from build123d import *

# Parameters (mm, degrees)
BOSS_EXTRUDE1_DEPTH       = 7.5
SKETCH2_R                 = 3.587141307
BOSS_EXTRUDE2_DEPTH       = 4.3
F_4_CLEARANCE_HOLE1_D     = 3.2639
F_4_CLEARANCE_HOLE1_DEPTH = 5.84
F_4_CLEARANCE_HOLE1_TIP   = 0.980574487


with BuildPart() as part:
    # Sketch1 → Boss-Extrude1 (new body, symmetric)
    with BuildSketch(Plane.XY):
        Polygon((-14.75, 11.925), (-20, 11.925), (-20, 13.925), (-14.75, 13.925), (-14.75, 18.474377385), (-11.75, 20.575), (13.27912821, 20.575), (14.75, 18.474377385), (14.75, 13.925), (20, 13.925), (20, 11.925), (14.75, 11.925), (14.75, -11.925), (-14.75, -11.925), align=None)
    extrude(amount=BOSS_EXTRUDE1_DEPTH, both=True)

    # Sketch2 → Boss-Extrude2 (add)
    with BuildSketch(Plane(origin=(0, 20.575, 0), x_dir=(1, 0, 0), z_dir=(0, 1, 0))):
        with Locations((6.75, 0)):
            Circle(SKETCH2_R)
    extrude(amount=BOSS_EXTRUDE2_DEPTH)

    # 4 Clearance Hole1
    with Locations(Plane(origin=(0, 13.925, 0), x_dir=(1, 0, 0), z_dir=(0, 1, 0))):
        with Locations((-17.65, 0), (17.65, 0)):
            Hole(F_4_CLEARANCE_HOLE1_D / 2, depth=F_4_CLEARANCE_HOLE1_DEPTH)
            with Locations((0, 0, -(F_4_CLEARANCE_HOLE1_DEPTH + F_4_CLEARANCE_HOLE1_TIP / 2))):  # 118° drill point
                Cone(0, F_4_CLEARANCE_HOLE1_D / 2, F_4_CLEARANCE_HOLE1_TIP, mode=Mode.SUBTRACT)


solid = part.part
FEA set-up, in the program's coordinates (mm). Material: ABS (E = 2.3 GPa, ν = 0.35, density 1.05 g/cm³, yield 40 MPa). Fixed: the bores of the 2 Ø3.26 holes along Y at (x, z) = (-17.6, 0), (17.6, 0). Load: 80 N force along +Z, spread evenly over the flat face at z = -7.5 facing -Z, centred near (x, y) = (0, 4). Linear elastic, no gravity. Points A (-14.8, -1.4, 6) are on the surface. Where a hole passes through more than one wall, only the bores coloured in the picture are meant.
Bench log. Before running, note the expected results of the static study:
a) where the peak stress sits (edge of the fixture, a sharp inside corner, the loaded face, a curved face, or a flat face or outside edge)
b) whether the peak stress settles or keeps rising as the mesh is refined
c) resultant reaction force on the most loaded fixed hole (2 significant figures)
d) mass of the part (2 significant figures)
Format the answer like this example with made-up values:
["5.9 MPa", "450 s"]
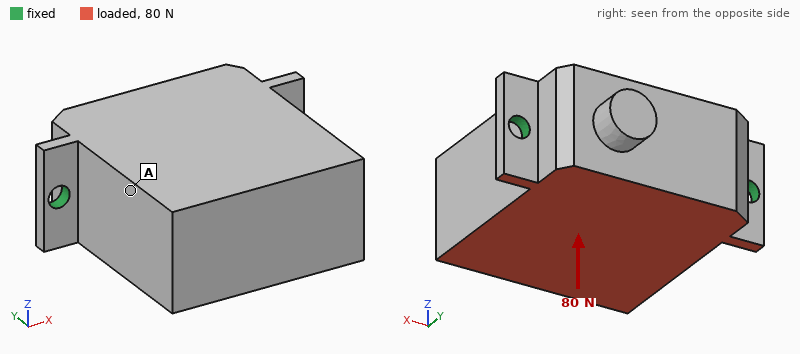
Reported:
["edge of the fixture", "keeps rising", "40 N", "16 g"]
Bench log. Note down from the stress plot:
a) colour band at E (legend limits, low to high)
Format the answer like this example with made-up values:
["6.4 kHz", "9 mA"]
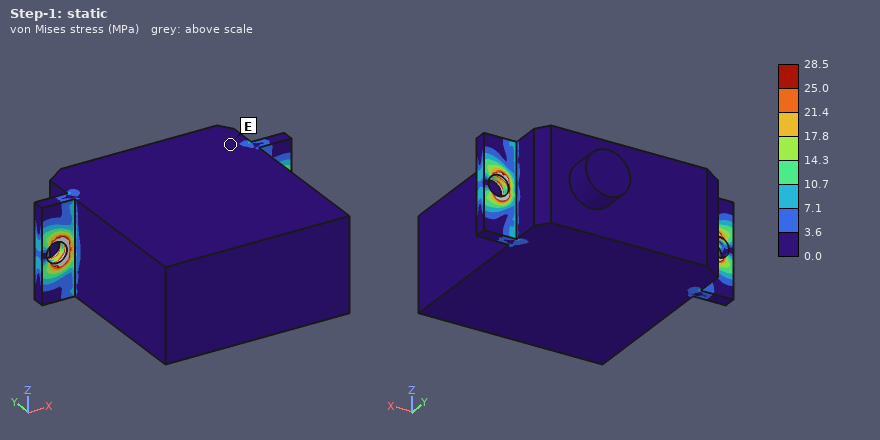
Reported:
["0.0 to 3.6 MPa"]
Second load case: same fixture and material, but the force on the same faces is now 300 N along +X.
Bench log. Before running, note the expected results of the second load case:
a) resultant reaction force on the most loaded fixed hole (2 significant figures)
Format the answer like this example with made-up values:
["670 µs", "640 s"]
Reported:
["180 N"]
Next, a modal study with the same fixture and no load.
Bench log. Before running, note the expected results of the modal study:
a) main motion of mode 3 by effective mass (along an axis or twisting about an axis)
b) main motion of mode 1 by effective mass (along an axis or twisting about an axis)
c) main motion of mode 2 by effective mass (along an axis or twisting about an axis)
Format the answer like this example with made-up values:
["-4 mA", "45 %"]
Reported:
["along Y", "along Z", "along X"]
